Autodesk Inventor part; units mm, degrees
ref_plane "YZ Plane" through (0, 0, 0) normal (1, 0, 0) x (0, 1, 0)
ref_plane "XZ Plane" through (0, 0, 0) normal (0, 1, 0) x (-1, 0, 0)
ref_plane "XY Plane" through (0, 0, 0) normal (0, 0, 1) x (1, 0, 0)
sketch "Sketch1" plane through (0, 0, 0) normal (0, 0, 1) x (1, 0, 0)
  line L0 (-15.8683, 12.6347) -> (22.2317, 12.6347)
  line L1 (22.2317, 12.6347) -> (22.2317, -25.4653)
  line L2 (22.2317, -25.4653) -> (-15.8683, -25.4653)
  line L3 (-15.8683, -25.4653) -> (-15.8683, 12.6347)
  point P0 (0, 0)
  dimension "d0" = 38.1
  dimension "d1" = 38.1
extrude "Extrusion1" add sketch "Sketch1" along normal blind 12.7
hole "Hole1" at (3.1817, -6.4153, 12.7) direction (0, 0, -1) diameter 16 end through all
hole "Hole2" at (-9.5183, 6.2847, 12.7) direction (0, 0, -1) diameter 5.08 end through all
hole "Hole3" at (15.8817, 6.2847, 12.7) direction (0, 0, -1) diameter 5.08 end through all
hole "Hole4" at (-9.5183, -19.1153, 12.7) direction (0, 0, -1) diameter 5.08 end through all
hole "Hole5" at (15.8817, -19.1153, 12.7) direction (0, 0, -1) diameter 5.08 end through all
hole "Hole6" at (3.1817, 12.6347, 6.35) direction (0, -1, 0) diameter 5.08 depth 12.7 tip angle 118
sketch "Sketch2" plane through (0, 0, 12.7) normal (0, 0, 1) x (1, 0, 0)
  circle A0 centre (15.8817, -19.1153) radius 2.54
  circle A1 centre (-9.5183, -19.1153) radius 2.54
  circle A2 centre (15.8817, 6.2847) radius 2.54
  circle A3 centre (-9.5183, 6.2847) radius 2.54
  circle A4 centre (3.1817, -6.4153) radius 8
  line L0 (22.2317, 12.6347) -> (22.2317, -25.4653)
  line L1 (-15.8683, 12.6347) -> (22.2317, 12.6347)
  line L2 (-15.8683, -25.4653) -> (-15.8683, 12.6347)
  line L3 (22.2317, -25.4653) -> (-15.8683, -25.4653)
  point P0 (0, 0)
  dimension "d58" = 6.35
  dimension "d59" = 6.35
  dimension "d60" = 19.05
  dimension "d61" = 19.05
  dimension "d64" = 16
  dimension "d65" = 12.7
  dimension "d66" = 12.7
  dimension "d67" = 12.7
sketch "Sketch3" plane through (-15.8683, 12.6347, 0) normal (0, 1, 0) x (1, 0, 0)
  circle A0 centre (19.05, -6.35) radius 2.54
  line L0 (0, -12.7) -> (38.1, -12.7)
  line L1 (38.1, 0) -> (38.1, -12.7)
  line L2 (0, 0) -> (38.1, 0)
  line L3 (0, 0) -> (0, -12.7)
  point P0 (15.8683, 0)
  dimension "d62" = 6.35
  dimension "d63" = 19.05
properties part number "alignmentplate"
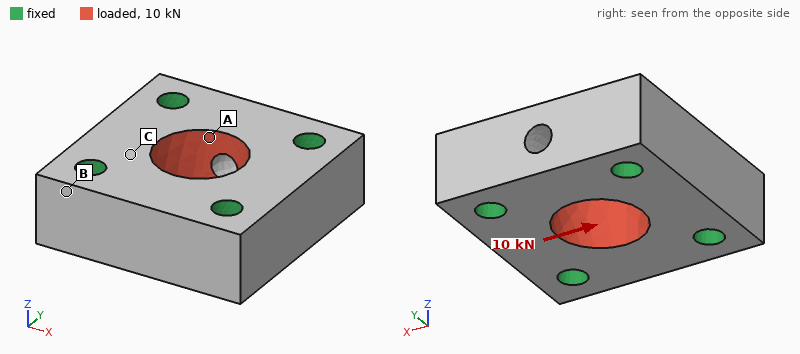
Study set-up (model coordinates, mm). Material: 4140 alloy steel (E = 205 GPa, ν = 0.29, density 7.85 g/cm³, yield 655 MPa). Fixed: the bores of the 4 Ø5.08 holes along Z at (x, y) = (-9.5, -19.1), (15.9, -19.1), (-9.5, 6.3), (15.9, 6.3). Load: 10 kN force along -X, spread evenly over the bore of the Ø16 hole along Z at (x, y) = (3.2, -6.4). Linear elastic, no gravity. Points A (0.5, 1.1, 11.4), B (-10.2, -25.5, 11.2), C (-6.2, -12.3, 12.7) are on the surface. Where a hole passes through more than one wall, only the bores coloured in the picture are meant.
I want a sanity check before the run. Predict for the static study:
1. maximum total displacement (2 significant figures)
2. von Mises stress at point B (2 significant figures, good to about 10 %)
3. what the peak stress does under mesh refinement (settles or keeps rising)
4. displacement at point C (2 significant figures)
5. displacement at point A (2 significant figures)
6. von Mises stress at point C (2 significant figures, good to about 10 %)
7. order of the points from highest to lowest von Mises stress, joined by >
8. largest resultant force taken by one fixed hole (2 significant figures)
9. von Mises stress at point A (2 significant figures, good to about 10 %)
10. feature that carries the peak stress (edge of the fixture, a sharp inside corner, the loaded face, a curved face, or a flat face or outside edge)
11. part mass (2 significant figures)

1.7 µm
5.0 MPa
keeps rising
0.98 µm
0.97 µm
18 MPa
A > C > B
2.7 kN
30 MPa
edge of the fixture
110 g
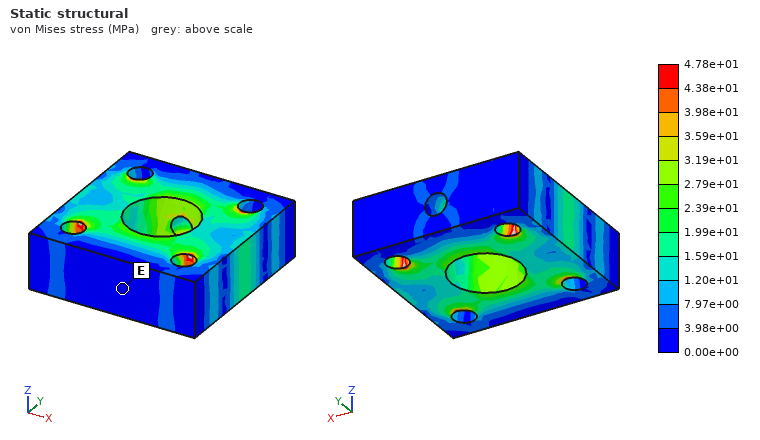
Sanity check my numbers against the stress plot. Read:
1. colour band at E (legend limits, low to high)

0.00e+00 to 3.98e+00 MPa
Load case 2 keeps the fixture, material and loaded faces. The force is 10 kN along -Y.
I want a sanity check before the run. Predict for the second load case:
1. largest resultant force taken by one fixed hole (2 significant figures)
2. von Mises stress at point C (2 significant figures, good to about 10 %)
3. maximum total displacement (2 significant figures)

2.7 kN
20 MPa
1.7 µm
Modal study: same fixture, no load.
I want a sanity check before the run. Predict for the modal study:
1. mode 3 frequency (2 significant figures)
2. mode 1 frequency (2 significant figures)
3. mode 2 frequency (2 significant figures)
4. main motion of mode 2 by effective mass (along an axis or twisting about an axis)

58 kHz
48 kHz
55 kHz
along Z
